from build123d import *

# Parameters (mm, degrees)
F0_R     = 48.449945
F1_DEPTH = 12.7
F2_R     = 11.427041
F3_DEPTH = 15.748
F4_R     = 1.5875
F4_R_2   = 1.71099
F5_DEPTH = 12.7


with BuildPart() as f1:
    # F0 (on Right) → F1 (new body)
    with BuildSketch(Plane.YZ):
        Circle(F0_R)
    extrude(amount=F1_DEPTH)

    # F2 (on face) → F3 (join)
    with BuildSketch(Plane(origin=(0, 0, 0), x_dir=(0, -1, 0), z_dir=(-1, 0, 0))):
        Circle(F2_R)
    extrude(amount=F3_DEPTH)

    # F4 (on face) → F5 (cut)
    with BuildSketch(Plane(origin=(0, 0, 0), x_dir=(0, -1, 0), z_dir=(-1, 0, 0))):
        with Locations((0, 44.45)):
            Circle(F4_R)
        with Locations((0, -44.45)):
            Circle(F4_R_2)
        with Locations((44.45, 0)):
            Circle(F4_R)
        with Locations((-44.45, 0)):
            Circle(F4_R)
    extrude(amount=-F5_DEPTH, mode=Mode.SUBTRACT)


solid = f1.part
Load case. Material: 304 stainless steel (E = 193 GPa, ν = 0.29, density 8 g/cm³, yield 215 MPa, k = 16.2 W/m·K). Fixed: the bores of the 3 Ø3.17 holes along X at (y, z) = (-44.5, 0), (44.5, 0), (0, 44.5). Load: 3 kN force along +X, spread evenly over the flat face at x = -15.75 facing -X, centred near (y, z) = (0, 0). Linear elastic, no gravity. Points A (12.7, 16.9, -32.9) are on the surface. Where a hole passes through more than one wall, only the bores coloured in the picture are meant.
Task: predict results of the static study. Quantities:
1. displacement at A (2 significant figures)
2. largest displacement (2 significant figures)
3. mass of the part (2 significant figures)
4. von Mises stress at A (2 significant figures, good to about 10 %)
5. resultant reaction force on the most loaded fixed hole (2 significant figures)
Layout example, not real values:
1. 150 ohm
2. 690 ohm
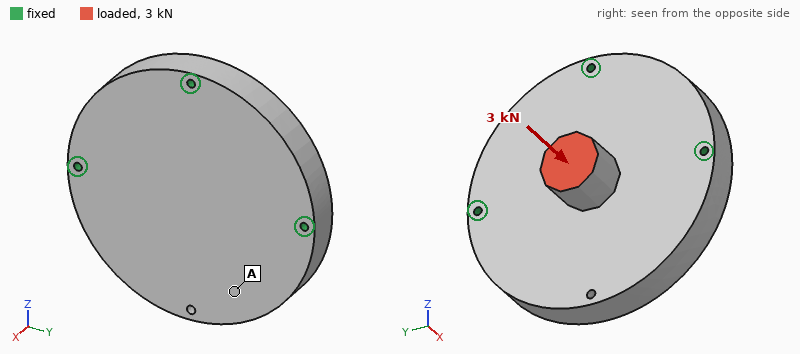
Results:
1. 11 µm
2. 15 µm
3. 800 g
4. 8.6 MPa
5. 1.2 kN
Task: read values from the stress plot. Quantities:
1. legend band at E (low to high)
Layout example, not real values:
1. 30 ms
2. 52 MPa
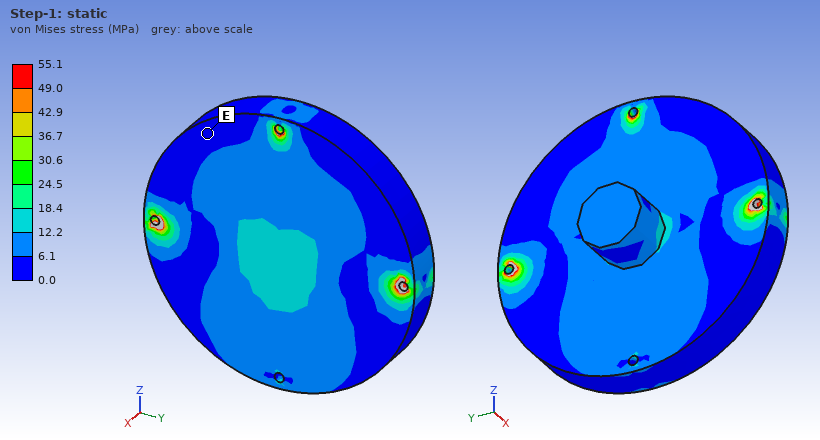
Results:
1. 0.0 to 6.1 MPa
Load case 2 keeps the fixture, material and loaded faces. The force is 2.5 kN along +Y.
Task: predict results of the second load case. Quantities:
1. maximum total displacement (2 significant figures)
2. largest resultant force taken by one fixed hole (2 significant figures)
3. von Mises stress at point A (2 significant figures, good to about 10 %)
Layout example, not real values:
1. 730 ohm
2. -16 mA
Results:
1. 8.4 µm
2. 1.2 kN
3. 3.4 MPa
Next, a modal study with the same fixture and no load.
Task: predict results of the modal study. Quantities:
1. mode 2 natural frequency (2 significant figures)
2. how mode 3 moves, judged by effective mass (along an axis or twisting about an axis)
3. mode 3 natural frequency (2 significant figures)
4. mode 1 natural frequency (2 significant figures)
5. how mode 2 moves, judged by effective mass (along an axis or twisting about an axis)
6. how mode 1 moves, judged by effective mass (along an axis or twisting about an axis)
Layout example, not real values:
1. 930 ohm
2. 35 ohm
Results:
1. 8100 Hz
2. twisting about Z
3. 8600 Hz
4. 3100 Hz
5. along X
6. along X
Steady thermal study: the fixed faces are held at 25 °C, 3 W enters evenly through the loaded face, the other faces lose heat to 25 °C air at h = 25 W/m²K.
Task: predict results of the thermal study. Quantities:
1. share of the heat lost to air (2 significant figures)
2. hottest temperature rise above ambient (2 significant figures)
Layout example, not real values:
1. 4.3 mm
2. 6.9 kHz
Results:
1. 39 %
2. 12 K
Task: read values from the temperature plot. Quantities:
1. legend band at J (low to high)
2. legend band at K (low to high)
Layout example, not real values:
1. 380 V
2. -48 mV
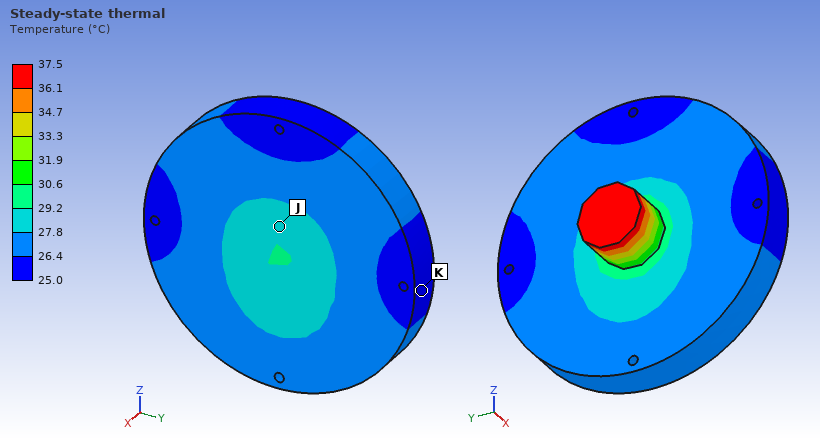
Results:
1. 27.8 to 29.2 °C
2. 25.0 to 26.4 °C
